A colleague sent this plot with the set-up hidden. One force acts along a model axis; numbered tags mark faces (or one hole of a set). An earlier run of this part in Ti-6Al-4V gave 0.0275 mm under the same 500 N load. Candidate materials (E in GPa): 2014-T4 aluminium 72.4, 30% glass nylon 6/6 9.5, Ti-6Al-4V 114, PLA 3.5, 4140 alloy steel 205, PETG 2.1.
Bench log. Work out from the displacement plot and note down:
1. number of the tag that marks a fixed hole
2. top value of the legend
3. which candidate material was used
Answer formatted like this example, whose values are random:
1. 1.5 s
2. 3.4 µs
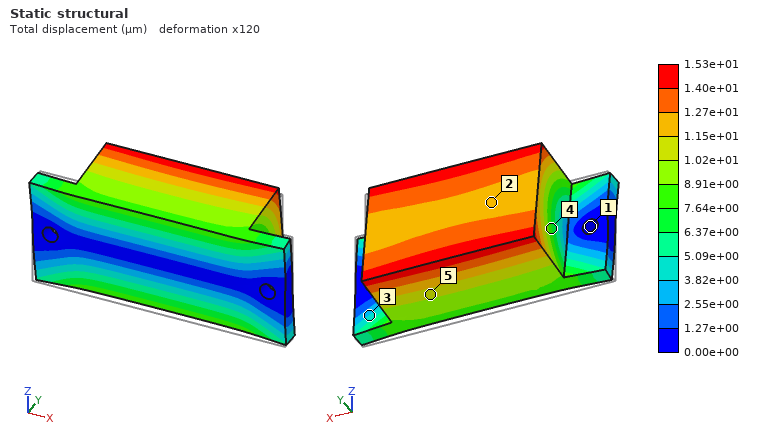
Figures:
1. 1
2. 1.53e+01 µm
3. 4140 alloy steel
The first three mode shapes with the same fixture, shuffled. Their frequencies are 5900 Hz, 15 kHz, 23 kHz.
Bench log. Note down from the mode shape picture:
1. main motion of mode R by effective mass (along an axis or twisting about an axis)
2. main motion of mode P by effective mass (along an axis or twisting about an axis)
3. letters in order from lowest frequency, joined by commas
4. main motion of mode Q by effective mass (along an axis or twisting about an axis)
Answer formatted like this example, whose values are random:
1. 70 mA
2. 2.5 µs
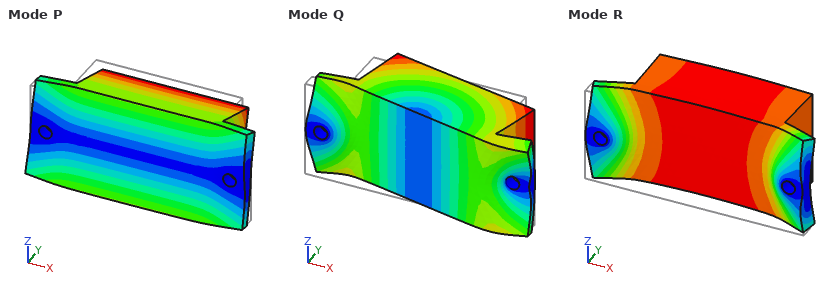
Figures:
1. along Y
2. along Z
3. P, R, Q
4. along X
